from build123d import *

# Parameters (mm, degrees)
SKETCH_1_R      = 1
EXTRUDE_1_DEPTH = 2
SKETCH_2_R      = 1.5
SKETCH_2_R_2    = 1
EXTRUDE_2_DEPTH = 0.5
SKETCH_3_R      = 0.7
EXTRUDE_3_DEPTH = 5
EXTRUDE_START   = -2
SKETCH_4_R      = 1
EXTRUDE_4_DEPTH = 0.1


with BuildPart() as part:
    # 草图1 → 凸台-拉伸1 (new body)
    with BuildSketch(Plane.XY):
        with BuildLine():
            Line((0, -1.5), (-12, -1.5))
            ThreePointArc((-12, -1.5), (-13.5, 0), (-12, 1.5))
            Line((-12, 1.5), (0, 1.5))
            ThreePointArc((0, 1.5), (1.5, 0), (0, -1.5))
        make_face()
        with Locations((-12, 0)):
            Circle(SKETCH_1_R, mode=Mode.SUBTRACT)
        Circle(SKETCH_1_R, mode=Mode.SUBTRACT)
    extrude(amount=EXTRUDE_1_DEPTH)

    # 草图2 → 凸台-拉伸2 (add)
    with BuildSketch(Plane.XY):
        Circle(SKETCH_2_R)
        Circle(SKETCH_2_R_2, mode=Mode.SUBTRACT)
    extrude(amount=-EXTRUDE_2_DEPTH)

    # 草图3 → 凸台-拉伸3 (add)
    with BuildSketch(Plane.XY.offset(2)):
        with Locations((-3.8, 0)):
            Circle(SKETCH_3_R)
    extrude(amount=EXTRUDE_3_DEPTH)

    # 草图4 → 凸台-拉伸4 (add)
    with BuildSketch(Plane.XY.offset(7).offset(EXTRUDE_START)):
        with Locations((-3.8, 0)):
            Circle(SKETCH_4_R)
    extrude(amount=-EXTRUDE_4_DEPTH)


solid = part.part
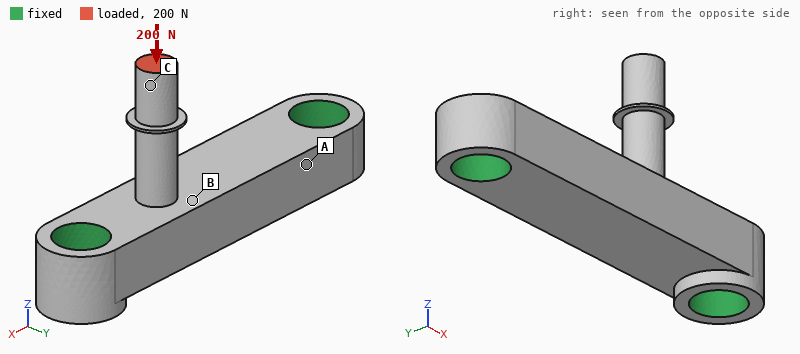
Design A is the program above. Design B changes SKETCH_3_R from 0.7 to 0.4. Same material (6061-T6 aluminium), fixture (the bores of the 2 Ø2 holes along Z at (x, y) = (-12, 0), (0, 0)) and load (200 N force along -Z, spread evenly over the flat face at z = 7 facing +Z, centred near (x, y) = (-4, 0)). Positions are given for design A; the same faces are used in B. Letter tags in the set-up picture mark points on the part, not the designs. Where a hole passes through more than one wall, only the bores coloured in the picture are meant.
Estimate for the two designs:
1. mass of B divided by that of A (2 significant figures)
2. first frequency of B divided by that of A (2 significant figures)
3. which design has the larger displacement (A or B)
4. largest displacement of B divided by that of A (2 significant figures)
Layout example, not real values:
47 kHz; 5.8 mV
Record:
0.94; 0.64; B; 1.9
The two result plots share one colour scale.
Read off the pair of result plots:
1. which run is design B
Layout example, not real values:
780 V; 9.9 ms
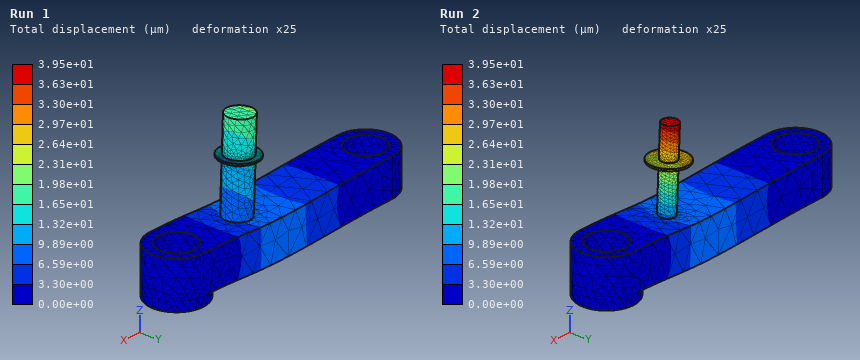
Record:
Run 2
